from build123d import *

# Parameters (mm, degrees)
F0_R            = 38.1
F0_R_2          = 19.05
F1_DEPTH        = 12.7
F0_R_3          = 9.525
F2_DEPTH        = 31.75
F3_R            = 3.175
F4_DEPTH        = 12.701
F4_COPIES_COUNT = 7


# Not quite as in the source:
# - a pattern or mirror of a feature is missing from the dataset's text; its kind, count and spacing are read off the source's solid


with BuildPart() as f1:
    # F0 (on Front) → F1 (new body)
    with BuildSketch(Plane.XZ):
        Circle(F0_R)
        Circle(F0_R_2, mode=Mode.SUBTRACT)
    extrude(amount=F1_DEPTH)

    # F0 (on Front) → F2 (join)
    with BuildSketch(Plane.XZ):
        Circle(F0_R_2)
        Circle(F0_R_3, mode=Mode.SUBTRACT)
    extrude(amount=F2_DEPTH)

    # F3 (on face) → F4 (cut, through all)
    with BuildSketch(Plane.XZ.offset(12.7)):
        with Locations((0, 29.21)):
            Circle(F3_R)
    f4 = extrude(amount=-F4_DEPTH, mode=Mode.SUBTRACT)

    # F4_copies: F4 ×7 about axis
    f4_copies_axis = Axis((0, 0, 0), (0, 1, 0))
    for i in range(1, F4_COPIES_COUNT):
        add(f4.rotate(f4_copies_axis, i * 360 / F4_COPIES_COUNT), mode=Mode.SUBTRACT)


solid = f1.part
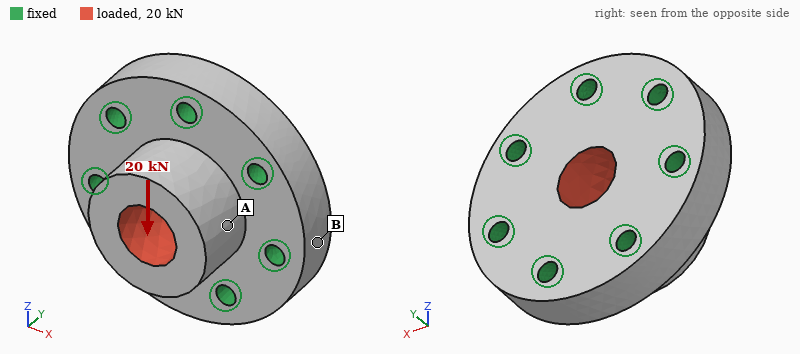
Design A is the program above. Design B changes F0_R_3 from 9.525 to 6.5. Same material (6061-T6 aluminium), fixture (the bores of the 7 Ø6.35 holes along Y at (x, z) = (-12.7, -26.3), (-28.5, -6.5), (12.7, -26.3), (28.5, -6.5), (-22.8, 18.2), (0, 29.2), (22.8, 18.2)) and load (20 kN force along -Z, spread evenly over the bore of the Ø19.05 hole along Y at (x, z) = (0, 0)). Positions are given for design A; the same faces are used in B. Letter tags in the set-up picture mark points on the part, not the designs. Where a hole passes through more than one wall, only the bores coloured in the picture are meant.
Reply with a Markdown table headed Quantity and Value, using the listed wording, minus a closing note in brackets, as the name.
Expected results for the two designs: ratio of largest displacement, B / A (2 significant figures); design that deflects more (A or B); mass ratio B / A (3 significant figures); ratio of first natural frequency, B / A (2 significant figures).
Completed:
| Quantity | Value |
|---|---|
| ratio of largest displacement, B / A | 0.90 |
| design that deflects more | A |
| mass ratio B / A | 1.07 |
| ratio of first natural frequency, B / A | 0.98 |
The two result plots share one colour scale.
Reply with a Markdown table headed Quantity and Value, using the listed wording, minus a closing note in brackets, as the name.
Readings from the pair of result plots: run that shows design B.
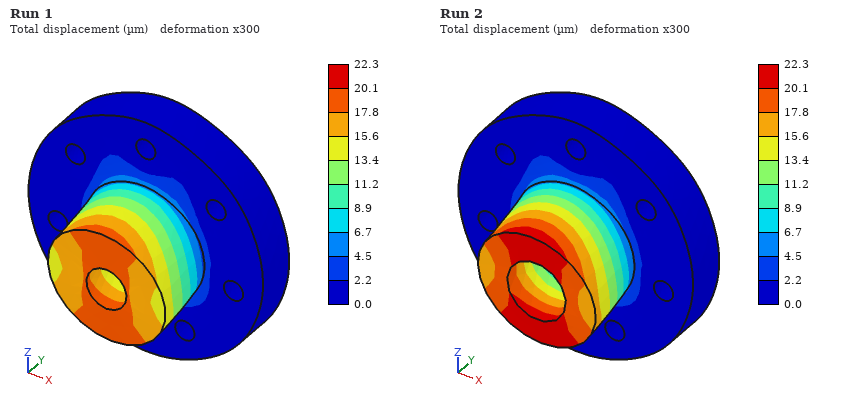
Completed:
| Quantity | Value |
|---|---|
| run that shows design B | Run 1 |
